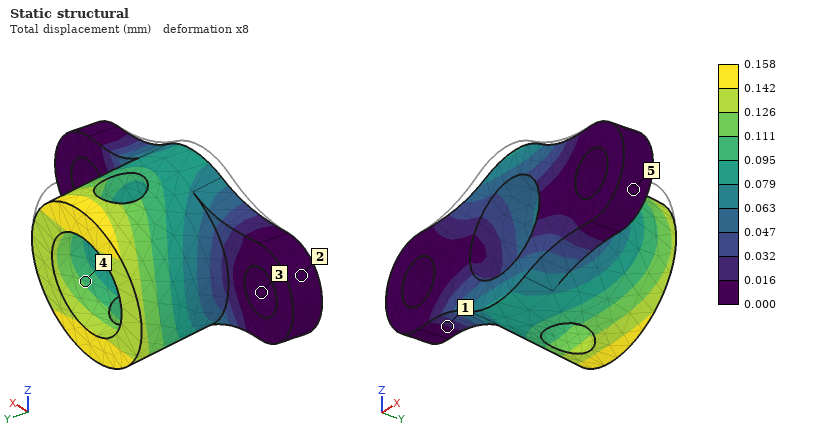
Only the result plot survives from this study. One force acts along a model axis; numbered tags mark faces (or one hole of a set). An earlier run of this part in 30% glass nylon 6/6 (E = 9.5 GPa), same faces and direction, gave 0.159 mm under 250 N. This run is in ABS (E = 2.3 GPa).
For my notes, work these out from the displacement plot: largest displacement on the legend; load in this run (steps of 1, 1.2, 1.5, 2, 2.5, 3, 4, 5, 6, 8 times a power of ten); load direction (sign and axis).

0.158 mm
60 N
-Z
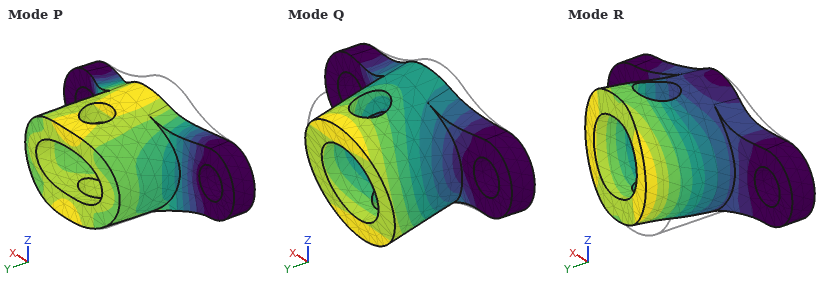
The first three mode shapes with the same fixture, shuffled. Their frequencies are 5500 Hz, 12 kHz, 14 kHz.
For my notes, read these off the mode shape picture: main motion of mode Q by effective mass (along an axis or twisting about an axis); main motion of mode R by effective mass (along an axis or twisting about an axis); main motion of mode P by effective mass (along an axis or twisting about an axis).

along Z
along X
along Y
